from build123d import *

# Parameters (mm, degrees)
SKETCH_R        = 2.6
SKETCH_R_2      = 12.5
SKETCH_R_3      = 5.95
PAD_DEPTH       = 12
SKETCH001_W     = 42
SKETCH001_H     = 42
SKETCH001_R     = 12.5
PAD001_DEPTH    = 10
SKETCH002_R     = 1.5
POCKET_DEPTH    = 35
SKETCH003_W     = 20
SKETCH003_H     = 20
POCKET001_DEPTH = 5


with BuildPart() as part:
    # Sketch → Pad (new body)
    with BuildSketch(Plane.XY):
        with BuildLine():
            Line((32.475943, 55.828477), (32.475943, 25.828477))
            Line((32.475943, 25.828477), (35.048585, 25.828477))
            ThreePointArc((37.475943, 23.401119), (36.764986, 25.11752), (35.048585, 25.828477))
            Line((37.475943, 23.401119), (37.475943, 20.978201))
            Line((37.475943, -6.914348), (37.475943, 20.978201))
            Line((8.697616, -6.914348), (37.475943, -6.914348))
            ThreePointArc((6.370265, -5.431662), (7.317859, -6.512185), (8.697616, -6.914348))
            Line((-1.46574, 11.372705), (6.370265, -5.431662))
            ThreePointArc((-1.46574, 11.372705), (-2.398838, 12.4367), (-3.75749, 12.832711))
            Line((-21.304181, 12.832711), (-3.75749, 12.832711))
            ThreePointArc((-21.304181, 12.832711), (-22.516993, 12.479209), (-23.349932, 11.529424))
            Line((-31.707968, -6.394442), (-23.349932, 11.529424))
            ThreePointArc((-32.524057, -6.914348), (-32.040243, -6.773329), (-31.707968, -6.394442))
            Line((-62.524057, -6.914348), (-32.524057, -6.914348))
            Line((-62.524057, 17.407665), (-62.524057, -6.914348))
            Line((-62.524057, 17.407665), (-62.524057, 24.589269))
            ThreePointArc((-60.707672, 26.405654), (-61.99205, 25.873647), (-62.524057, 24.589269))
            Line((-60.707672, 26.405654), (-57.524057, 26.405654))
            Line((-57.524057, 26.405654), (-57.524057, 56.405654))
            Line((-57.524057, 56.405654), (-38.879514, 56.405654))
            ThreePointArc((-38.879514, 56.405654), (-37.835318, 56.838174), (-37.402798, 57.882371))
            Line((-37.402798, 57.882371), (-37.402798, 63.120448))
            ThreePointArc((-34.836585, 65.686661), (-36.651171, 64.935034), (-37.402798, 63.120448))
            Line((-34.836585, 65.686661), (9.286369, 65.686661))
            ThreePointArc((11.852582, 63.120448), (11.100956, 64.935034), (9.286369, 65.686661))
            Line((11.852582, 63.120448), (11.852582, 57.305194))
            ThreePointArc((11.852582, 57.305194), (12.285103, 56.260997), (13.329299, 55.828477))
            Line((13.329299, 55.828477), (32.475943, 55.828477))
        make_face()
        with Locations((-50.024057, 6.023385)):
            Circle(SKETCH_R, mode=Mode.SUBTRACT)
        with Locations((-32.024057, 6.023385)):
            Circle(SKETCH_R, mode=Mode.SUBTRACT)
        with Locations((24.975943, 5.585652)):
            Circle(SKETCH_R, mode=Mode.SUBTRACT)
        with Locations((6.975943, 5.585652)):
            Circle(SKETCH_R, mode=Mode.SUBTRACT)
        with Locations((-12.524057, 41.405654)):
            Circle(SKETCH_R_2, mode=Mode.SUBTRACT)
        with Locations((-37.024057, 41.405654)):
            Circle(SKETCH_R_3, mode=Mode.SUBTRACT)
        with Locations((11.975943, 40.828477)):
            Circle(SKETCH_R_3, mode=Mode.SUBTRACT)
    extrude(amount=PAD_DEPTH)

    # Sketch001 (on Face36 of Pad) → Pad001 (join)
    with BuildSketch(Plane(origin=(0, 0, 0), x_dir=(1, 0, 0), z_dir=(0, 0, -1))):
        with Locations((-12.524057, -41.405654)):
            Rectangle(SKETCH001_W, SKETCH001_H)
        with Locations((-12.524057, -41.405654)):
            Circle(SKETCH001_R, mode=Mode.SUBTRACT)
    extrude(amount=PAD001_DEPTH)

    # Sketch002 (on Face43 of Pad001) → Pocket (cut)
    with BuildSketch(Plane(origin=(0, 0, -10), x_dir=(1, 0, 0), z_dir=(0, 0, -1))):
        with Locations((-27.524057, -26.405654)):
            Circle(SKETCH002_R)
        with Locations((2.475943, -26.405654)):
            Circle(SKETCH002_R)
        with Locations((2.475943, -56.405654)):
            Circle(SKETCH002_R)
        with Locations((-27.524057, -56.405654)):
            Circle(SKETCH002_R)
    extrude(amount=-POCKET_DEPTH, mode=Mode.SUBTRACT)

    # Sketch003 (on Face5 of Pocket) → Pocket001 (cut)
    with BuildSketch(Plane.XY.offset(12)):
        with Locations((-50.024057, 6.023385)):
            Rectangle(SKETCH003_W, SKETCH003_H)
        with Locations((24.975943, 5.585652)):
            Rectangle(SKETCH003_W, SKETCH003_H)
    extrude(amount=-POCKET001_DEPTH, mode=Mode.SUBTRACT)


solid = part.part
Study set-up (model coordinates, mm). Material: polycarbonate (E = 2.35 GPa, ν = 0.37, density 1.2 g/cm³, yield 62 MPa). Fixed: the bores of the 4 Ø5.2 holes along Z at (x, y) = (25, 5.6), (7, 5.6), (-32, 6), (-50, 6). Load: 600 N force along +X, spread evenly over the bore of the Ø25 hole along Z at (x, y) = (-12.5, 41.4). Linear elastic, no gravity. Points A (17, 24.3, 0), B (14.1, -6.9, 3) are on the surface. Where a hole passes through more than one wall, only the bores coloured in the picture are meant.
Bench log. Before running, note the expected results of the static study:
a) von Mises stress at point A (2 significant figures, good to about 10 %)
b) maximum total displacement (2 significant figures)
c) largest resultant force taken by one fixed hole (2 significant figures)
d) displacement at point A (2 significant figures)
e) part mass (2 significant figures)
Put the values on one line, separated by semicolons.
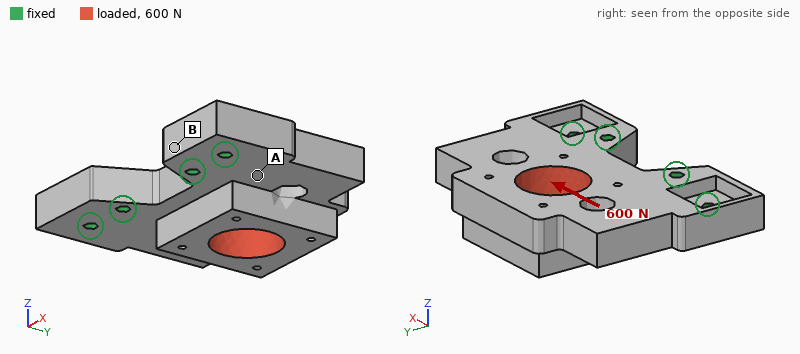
1.5 MPa; 88 µm; 270 N; 28 µm; 83 g
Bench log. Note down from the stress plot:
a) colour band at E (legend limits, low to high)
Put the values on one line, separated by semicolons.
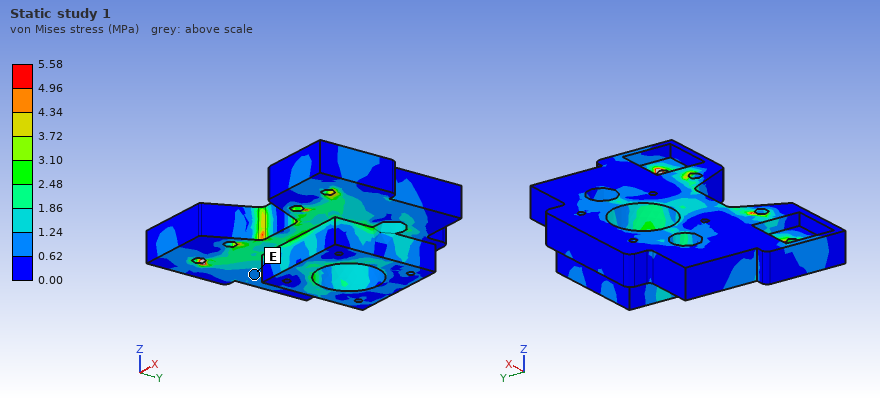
0.62 to 1.24 MPa
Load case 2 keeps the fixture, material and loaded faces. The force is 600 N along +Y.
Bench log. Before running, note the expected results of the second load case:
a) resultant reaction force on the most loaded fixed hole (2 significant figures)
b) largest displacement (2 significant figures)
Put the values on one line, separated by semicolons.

200 N; 0.17 mm
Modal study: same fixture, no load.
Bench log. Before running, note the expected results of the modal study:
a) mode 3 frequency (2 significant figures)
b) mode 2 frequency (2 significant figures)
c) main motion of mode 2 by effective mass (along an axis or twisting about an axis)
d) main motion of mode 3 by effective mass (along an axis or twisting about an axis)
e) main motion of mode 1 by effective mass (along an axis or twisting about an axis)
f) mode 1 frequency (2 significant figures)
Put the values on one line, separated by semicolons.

2200 Hz; 1400 Hz; twisting about Y; along X; along Z; 630 Hz
